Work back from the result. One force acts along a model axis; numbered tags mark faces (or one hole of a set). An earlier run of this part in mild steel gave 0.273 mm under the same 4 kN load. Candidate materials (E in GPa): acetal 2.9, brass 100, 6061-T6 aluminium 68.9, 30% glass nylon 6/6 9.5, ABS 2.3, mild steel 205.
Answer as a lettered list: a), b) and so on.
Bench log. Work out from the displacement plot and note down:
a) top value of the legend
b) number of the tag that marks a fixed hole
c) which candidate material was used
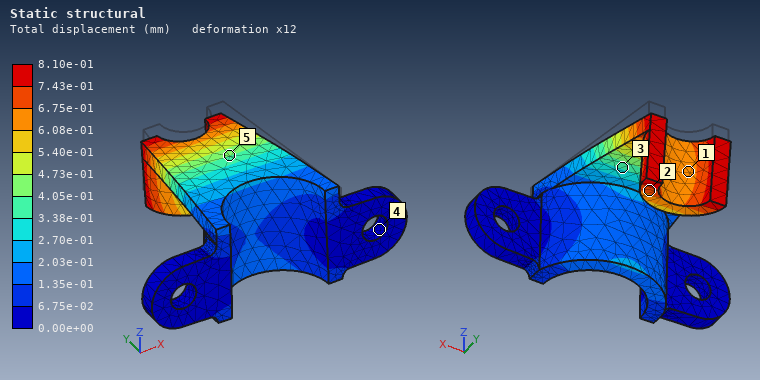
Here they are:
a) 8.10e-01 mm
b) 4
c) 6061-T6 aluminium
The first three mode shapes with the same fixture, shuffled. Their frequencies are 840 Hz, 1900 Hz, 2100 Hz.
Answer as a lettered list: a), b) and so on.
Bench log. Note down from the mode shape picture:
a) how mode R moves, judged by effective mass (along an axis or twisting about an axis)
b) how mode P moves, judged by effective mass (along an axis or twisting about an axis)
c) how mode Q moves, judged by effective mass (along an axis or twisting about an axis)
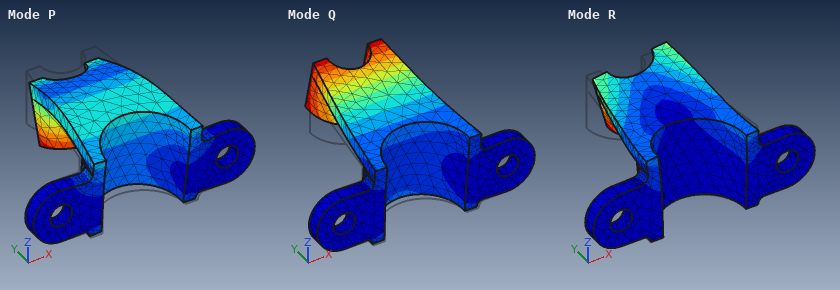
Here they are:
a) along X
b) along Y
c) along Z
